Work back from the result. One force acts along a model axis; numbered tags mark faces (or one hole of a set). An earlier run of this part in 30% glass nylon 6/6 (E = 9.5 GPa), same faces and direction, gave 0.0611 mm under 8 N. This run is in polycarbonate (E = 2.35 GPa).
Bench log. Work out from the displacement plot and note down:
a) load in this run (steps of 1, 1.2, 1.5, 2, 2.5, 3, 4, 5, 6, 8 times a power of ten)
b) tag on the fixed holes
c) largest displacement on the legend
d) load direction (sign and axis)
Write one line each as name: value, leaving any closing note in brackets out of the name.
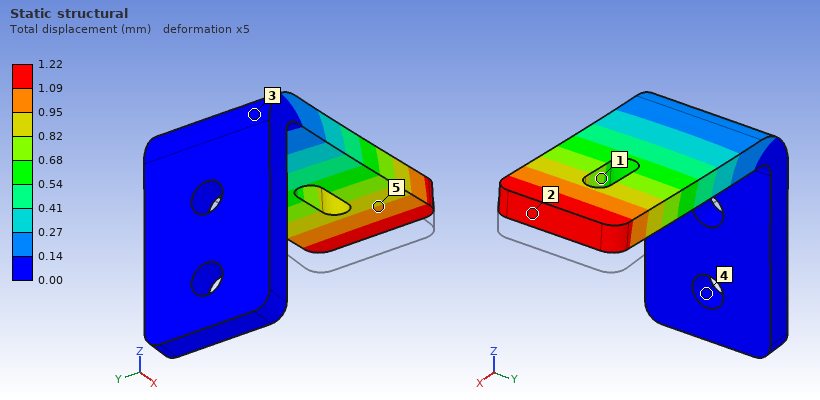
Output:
load in this run: 40 N
tag on the fixed holes: 4
largest displacement on the legend: 1.22 mm
load direction: +Z
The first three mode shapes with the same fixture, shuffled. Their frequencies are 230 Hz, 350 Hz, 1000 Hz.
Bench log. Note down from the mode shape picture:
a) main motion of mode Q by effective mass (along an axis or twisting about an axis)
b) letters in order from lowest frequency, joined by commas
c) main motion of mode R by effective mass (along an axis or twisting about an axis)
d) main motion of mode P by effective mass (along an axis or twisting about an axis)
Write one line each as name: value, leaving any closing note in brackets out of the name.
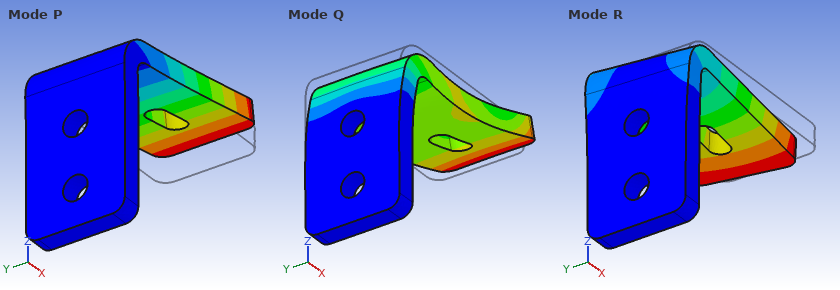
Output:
main motion of mode Q by effective mass: along X
letters in order from lowest frequency, joined by commas: P, R, Q
main motion of mode R by effective mass: along Y
main motion of mode P by effective mass: along Z
